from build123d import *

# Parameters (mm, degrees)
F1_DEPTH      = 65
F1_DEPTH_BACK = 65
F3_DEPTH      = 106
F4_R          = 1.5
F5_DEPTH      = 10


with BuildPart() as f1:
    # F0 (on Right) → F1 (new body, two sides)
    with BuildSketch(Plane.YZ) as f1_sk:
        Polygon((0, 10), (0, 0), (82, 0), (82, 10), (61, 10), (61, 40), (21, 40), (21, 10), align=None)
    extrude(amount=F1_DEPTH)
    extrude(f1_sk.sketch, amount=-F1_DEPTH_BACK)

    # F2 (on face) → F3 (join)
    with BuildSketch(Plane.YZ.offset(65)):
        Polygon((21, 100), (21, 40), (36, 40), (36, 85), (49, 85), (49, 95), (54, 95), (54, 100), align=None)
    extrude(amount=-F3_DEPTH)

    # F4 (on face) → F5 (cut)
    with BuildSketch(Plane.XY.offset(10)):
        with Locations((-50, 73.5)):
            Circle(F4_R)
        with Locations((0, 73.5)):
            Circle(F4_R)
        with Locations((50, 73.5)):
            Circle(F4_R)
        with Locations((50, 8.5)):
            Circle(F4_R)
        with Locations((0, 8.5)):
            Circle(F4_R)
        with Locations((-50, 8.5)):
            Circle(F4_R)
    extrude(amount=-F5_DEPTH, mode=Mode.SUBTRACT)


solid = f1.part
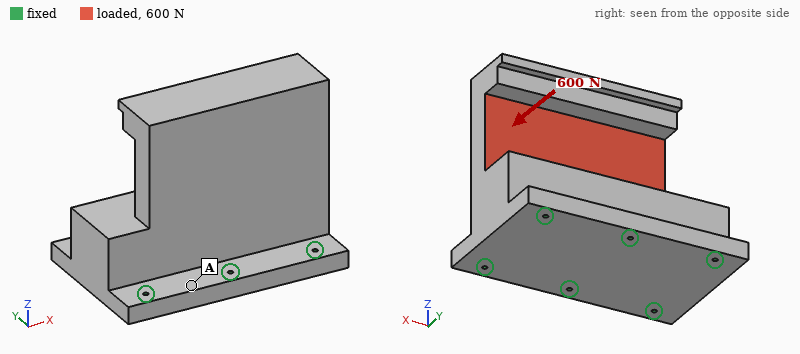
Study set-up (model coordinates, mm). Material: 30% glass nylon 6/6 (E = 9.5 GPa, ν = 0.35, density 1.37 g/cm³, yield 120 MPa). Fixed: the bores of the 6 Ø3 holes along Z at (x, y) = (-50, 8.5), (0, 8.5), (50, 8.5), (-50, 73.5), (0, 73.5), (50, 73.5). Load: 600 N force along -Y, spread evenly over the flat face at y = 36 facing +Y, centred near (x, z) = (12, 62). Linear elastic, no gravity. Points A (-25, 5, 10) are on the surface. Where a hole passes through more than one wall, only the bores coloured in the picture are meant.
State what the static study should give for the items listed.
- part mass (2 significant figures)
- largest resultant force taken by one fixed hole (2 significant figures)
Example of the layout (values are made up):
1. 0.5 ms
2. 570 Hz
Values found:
1. 520 g
2. 260 N
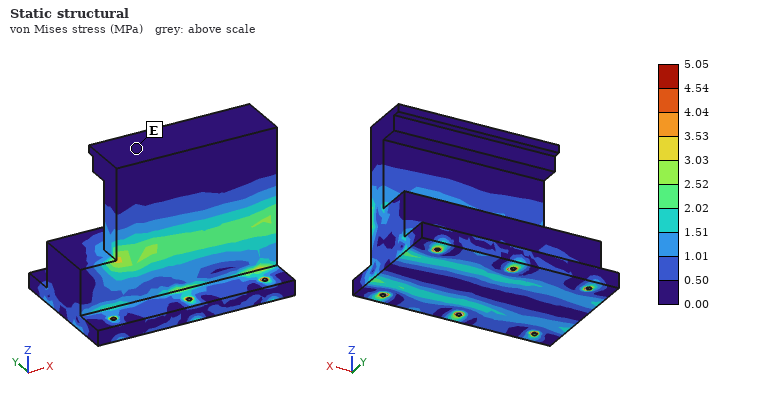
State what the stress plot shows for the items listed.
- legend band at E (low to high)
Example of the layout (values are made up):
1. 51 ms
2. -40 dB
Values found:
1. 0.00 to 0.50 MPa
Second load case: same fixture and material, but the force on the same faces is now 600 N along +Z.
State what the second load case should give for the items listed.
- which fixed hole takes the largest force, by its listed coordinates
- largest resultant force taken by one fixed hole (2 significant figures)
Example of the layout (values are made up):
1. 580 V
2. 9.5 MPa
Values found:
1. (50, 8.5)
2. 150 N
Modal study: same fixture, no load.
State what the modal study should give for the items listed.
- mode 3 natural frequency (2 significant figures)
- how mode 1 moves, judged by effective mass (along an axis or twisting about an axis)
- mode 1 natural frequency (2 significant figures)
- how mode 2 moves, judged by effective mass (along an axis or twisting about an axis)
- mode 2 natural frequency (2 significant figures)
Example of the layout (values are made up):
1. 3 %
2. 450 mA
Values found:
1. 1800 Hz
2. along Y
3. 900 Hz
4. along X
5. 1500 Hz
